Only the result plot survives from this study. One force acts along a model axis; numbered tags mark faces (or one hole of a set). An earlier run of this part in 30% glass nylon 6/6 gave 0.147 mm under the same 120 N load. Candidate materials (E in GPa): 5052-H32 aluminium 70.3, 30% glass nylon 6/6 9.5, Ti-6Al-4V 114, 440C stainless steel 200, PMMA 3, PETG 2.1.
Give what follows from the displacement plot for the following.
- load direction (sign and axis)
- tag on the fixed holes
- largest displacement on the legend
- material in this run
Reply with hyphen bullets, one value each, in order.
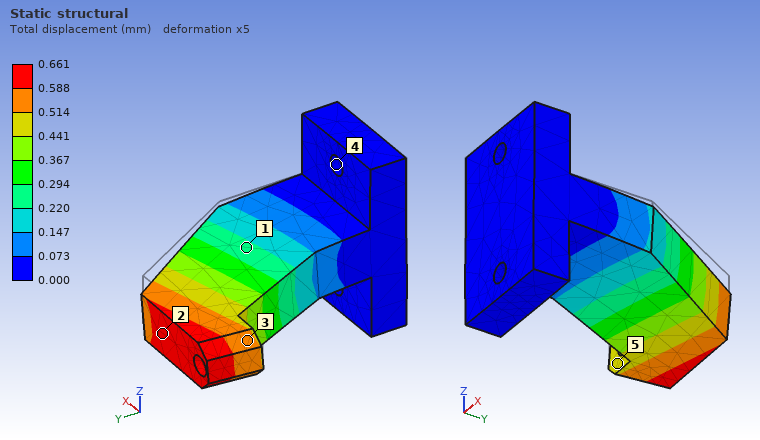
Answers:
- -Z
- 4
- 0.661 mm
- PETG
